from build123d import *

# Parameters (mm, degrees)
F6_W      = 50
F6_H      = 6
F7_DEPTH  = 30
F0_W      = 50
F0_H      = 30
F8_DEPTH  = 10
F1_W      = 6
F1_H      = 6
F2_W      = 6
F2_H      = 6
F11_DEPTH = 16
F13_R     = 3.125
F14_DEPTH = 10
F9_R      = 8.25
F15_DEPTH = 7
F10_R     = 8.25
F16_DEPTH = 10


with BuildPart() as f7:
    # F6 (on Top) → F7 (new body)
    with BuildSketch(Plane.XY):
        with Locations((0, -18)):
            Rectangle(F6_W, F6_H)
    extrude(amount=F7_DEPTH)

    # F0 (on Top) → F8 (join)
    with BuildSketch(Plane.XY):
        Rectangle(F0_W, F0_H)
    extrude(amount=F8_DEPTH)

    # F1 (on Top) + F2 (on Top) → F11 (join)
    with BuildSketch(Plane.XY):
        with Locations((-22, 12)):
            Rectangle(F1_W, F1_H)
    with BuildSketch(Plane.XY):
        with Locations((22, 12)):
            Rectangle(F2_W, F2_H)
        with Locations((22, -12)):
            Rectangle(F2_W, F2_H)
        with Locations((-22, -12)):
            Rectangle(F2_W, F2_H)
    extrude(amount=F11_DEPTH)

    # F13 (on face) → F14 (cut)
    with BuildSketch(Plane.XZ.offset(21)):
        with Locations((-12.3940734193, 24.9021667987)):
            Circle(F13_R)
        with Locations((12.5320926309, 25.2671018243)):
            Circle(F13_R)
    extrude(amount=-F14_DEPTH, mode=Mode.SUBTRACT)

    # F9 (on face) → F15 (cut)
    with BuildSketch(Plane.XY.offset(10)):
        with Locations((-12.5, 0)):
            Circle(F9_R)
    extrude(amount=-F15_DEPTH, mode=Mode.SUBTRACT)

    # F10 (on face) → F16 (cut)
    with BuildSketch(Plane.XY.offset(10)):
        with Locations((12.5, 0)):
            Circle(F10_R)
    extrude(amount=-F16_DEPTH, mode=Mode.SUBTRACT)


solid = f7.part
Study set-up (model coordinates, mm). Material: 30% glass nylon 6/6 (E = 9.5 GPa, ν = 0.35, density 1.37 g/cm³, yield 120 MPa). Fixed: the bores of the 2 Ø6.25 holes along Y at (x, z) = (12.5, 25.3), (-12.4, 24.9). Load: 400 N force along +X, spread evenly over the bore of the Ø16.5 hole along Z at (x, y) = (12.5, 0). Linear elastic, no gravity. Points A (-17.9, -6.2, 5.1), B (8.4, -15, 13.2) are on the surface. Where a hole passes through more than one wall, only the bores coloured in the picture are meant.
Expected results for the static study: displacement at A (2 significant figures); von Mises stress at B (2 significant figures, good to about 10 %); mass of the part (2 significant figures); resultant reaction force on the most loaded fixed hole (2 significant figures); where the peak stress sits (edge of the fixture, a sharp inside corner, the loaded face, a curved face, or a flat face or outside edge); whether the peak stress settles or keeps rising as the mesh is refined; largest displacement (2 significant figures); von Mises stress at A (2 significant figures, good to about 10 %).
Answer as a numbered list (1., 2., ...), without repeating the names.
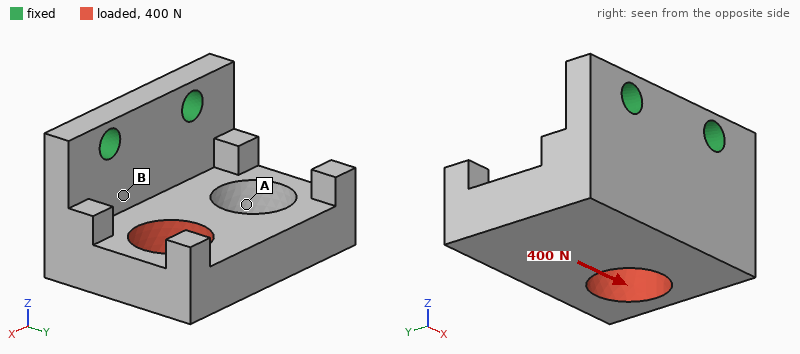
1. 0.066 mm
2. 9.4 MPa
3. 29 g
4. 390 N
5. edge of the fixture
6. keeps rising
7. 0.15 mm
8. 3.3 MPa
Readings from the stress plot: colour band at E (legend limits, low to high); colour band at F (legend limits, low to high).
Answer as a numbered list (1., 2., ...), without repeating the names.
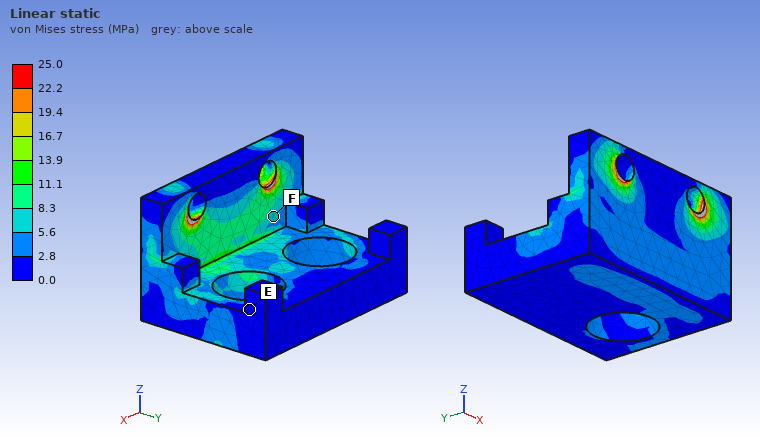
1. 0.0 to 2.8 MPa
2. 5.6 to 8.3 MPa
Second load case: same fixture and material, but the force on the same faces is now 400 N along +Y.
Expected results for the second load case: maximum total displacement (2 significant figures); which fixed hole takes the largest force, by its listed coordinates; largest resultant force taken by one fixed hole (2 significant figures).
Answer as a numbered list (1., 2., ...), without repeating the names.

1. 0.38 mm
2. (12.5, 25.3)
3. 350 N
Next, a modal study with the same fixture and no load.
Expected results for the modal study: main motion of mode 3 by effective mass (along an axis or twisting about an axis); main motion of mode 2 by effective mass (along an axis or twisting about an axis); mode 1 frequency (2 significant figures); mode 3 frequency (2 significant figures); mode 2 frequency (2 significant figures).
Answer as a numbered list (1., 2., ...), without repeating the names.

1. along Y
2. along X
3. 1200 Hz
4. 4100 Hz
5. 2100 Hz
